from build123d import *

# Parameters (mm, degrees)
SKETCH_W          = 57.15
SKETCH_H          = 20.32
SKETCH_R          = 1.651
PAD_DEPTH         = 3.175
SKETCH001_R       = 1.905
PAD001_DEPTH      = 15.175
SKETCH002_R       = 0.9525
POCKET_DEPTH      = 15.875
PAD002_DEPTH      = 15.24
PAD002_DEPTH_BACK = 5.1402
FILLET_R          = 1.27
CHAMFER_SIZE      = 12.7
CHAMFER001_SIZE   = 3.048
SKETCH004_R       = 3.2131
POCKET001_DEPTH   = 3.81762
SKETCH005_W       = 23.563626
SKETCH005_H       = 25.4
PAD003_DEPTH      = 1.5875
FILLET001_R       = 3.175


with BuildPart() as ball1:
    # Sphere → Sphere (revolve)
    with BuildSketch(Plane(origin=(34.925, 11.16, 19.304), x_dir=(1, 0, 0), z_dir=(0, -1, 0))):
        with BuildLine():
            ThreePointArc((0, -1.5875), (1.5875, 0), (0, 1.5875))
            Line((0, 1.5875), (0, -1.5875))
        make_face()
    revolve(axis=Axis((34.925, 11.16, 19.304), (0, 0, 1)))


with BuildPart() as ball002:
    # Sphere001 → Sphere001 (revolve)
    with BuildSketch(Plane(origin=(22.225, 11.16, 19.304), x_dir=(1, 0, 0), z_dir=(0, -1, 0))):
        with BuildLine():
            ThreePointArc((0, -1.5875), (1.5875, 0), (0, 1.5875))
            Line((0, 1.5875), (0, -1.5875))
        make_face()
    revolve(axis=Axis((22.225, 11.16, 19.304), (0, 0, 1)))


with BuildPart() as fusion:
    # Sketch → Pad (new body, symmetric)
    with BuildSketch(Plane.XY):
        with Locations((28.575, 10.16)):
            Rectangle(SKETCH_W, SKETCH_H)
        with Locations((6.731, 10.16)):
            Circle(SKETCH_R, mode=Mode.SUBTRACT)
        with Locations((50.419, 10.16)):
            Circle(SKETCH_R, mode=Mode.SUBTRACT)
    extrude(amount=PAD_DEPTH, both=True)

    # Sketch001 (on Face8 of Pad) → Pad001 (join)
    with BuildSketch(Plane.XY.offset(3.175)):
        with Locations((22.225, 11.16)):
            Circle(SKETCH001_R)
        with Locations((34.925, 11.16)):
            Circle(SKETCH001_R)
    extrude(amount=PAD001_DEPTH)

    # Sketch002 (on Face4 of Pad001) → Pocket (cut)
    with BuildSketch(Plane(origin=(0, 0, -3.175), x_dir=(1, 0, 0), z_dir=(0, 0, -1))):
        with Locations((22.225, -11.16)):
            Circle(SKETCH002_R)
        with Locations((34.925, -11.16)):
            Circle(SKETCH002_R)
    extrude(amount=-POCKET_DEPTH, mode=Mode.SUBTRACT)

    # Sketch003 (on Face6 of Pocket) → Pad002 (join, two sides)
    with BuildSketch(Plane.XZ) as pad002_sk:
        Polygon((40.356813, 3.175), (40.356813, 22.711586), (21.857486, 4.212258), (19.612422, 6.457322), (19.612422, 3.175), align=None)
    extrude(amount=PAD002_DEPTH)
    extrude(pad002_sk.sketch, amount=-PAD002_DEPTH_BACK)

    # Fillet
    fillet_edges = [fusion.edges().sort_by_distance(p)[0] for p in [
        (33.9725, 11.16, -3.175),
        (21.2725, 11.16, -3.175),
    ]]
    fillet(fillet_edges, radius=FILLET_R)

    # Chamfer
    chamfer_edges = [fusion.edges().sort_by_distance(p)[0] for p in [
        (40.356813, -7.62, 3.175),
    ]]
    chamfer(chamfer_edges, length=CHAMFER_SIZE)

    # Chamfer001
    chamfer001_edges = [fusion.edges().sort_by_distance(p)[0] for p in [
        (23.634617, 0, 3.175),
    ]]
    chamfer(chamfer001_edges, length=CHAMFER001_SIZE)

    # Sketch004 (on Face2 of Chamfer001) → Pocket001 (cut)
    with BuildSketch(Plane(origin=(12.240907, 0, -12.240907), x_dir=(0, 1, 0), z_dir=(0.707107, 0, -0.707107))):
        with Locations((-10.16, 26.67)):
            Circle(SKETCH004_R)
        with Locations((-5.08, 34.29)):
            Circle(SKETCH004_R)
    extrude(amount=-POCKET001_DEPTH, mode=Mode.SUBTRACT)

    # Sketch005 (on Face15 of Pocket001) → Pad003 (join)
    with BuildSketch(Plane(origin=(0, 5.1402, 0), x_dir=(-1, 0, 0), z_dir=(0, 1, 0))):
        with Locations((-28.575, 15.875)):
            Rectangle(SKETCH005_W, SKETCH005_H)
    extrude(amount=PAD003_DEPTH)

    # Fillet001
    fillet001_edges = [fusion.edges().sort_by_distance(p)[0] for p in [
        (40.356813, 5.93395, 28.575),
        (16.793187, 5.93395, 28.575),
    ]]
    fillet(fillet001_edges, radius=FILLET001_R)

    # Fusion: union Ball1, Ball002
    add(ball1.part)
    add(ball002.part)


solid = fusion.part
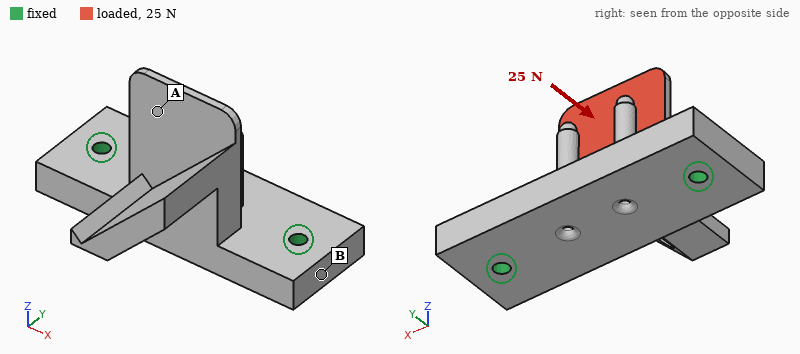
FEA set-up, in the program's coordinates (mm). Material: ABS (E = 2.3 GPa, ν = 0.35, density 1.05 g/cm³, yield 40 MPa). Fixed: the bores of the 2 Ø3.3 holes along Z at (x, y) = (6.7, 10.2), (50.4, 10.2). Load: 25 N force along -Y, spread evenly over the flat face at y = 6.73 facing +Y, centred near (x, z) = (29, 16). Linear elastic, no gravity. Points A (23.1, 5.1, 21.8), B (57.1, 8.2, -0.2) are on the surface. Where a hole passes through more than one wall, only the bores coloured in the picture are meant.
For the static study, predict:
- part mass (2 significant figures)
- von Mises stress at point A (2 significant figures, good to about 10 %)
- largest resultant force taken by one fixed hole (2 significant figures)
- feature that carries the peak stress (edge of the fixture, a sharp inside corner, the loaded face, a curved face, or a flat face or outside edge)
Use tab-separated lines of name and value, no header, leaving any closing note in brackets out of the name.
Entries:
part mass	12 g
von Mises stress at point A	1.8 MPa
largest resultant force taken by one fixed hole	13 N
feature that carries the peak stress	the loaded face
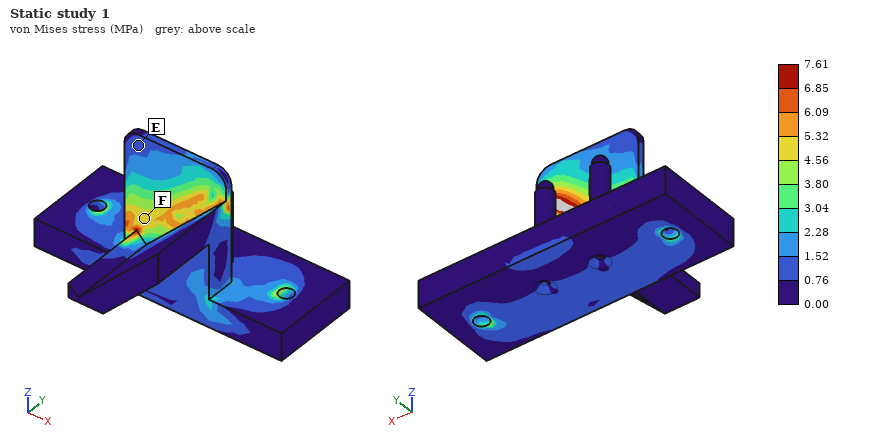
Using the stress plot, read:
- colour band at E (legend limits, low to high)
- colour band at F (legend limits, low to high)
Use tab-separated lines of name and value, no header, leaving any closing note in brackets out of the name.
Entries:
colour band at E	0.76 to 1.52 MPa
colour band at F	4.56 to 5.32 MPa
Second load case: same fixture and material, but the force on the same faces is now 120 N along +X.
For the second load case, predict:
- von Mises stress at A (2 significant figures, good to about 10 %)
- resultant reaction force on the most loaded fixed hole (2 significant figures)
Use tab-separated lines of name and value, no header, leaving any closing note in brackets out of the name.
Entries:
von Mises stress at A	0.59 MPa
resultant reaction force on the most loaded fixed hole	82 N
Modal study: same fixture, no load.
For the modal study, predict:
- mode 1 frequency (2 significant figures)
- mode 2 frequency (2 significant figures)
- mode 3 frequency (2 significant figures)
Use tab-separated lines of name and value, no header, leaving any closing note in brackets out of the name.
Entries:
mode 1 frequency	1200 Hz
mode 2 frequency	1800 Hz
mode 3 frequency	2400 Hz
